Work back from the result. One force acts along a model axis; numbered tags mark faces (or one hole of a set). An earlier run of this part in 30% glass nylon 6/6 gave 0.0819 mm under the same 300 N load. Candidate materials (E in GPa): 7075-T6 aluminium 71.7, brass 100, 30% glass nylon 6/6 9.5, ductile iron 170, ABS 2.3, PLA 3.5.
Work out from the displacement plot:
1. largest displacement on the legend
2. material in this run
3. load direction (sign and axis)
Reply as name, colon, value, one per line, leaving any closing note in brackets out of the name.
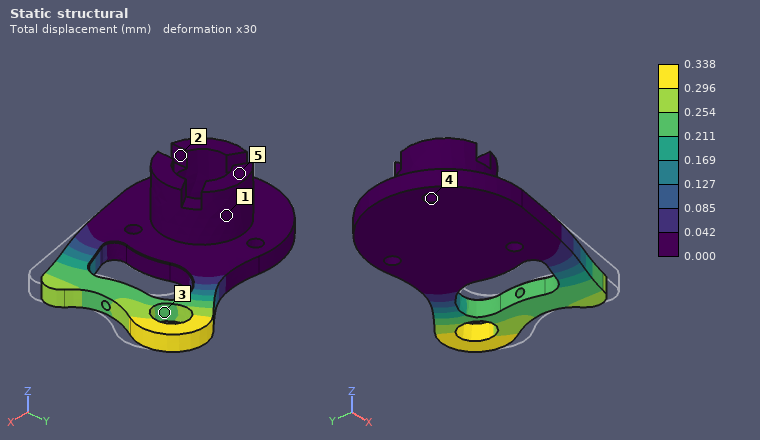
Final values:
largest displacement on the legend: 0.338 mm
material in this run: ABS
load direction: +Y
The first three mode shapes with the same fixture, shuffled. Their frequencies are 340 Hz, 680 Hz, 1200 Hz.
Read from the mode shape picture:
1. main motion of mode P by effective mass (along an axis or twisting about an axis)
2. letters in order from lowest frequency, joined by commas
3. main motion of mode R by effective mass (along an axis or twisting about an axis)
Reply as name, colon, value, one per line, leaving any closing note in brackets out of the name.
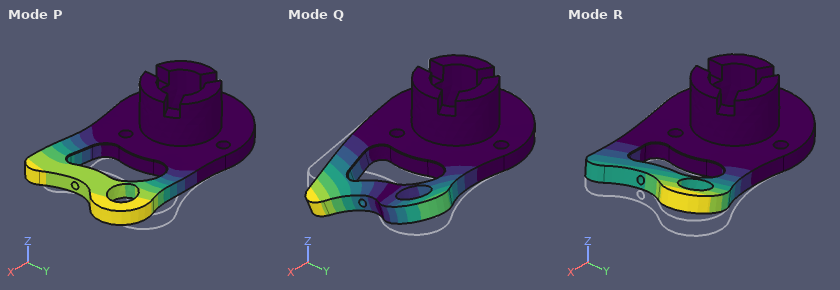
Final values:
main motion of mode P by effective mass: along Y
letters in order from lowest frequency, joined by commas: R, Q, P
main motion of mode R by effective mass: along Z
